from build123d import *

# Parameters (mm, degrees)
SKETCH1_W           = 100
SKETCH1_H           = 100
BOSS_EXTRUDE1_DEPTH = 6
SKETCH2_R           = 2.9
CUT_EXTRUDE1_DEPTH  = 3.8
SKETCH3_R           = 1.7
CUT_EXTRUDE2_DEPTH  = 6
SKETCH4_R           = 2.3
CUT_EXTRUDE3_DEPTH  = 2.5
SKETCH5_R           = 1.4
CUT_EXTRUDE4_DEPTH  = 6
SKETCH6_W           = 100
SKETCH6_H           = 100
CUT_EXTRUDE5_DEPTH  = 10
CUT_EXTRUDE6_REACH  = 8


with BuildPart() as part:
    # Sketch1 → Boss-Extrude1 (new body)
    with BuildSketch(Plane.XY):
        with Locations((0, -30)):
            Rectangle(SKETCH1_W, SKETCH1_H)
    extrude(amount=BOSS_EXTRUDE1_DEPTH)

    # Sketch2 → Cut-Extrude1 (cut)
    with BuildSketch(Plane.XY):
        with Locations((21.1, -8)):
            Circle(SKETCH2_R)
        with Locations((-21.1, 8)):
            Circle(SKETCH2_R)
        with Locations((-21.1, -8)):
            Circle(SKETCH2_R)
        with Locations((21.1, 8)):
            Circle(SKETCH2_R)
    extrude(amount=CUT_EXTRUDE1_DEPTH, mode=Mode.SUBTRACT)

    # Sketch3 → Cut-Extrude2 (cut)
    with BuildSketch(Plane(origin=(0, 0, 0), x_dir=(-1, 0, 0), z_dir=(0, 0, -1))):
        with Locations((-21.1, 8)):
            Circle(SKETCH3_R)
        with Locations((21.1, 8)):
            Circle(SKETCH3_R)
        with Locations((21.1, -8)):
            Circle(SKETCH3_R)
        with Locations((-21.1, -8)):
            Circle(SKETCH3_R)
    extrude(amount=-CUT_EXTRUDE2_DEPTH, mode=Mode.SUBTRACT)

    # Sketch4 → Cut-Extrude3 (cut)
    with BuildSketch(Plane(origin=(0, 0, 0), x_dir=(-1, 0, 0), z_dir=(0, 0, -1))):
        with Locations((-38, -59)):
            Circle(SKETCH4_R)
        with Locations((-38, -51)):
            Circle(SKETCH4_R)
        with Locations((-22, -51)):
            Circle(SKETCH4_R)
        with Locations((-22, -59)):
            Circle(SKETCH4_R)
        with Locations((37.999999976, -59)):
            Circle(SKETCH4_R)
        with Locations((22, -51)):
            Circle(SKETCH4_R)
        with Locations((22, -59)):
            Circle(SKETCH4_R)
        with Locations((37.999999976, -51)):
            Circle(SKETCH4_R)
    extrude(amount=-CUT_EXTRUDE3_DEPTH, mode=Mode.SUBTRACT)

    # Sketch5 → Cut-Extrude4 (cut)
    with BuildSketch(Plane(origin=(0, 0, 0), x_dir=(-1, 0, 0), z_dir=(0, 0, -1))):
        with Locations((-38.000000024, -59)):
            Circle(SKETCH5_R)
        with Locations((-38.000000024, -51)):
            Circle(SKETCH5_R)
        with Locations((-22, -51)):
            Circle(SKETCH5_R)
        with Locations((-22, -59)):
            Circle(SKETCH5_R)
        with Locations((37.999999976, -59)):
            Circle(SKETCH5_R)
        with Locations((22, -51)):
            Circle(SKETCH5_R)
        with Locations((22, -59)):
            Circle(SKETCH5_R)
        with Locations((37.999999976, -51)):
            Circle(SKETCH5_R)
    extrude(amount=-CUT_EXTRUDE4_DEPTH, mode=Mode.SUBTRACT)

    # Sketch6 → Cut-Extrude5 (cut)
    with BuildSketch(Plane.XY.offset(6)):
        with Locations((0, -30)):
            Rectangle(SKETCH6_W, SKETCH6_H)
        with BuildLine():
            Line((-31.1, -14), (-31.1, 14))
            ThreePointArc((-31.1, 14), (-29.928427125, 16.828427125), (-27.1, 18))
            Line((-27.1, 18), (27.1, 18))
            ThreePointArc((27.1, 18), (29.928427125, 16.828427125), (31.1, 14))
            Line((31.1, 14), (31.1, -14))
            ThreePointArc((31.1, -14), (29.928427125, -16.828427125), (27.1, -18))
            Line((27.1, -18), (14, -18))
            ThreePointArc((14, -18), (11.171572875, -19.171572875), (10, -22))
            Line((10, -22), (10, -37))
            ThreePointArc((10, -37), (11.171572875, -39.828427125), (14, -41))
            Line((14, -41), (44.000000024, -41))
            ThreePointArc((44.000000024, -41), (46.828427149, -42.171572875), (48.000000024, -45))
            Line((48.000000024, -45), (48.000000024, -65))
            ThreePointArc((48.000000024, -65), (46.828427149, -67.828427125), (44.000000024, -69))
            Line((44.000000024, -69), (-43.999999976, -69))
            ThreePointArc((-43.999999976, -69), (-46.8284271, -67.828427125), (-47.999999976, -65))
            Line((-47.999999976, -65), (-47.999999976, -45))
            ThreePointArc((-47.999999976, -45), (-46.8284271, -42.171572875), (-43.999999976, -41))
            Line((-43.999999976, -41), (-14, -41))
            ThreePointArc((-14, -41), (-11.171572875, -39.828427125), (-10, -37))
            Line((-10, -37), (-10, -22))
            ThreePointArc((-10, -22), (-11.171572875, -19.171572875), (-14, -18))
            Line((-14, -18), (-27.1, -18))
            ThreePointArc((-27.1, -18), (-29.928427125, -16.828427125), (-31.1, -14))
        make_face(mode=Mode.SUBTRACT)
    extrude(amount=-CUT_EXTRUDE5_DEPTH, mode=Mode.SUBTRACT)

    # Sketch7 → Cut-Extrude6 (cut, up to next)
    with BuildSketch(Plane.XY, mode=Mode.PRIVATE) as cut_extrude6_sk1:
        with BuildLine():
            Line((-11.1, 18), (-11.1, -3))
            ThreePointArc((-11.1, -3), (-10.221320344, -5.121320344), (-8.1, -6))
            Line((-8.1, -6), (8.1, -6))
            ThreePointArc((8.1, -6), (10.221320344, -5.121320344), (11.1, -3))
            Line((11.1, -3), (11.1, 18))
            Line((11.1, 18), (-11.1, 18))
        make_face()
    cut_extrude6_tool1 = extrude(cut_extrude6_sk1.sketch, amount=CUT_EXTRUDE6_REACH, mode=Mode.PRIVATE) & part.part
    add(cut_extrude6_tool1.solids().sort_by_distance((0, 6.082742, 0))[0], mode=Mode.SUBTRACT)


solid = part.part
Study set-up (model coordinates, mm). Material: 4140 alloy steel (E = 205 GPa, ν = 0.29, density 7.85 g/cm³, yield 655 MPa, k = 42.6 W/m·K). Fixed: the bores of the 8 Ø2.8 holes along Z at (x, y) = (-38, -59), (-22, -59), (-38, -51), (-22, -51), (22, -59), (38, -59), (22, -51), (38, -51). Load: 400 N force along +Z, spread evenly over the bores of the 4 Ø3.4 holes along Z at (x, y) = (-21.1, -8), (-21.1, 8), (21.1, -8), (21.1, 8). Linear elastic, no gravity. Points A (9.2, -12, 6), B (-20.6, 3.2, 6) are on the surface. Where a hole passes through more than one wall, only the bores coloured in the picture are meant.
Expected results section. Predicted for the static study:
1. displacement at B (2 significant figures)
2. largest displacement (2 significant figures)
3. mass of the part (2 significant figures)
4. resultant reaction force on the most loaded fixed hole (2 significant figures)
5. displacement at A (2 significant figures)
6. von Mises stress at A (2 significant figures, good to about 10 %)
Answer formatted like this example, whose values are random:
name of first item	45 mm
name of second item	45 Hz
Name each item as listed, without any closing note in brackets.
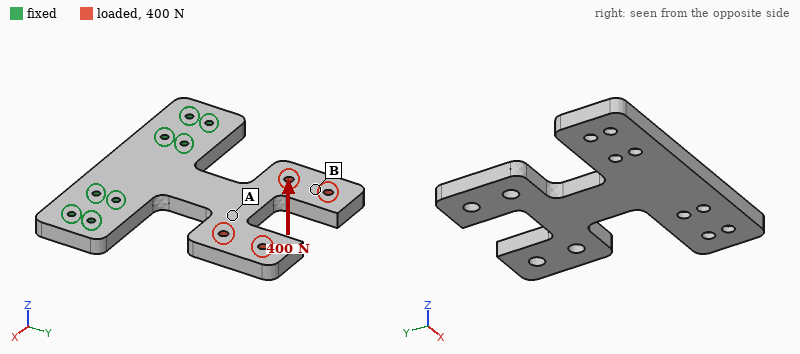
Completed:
displacement at B	0.28 mm
largest displacement	0.39 mm
mass of the part	220 g
resultant reaction force on the most loaded fixed hole	1.1 kN
displacement at A	0.17 mm
von Mises stress at A	36 MPa
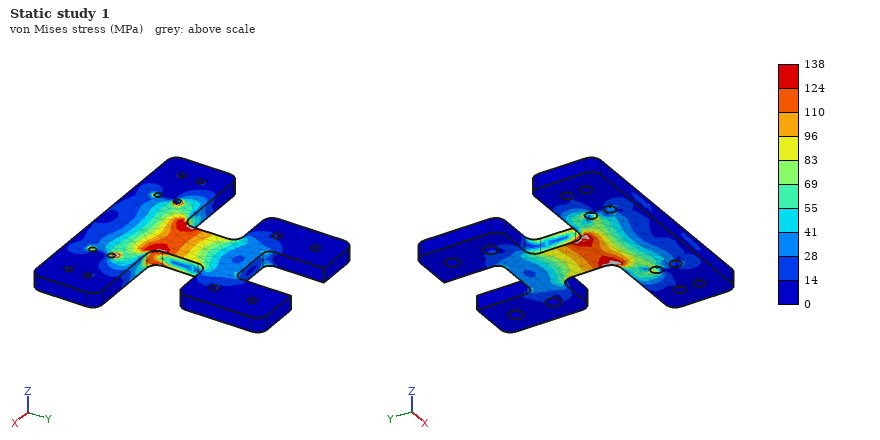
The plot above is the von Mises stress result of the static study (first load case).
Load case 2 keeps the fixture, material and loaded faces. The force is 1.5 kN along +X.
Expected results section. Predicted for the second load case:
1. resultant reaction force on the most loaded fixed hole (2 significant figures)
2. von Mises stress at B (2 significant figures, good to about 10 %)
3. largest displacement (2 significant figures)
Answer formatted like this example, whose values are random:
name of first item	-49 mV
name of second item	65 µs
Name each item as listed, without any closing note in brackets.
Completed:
resultant reaction force on the most loaded fixed hole	1.1 kN
von Mises stress at B	15 MPa
largest displacement	0.14 mm
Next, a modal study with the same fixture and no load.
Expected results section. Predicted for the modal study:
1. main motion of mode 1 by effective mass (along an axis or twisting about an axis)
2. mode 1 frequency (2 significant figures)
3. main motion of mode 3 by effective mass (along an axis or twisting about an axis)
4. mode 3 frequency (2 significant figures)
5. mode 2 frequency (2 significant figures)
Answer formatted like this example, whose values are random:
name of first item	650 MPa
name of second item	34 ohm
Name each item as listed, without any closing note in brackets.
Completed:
main motion of mode 1 by effective mass	along Z
mode 1 frequency	720 Hz
main motion of mode 3 by effective mass	along X
mode 3 frequency	2300 Hz
mode 2 frequency	1400 Hz
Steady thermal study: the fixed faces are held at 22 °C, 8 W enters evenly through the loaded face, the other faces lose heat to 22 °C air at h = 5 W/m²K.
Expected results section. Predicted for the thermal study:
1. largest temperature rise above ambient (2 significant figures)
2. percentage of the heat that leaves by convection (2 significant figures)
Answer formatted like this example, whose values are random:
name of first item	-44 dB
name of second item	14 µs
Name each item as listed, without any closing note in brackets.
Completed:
largest temperature rise above ambient	68 K
percentage of the heat that leaves by convection	21 %
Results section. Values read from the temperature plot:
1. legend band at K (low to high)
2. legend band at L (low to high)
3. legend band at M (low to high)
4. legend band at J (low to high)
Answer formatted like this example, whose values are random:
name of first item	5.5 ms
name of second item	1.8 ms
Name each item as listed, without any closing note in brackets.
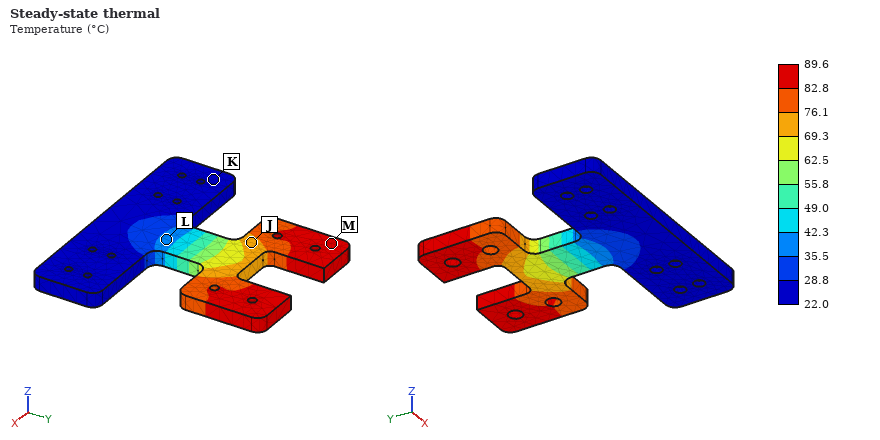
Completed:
legend band at K	22.0 to 28.8 °C
legend band at L	35.5 to 42.3 °C
legend band at M	82.8 to 89.6 °C
legend band at J	69.3 to 76.1 °C
